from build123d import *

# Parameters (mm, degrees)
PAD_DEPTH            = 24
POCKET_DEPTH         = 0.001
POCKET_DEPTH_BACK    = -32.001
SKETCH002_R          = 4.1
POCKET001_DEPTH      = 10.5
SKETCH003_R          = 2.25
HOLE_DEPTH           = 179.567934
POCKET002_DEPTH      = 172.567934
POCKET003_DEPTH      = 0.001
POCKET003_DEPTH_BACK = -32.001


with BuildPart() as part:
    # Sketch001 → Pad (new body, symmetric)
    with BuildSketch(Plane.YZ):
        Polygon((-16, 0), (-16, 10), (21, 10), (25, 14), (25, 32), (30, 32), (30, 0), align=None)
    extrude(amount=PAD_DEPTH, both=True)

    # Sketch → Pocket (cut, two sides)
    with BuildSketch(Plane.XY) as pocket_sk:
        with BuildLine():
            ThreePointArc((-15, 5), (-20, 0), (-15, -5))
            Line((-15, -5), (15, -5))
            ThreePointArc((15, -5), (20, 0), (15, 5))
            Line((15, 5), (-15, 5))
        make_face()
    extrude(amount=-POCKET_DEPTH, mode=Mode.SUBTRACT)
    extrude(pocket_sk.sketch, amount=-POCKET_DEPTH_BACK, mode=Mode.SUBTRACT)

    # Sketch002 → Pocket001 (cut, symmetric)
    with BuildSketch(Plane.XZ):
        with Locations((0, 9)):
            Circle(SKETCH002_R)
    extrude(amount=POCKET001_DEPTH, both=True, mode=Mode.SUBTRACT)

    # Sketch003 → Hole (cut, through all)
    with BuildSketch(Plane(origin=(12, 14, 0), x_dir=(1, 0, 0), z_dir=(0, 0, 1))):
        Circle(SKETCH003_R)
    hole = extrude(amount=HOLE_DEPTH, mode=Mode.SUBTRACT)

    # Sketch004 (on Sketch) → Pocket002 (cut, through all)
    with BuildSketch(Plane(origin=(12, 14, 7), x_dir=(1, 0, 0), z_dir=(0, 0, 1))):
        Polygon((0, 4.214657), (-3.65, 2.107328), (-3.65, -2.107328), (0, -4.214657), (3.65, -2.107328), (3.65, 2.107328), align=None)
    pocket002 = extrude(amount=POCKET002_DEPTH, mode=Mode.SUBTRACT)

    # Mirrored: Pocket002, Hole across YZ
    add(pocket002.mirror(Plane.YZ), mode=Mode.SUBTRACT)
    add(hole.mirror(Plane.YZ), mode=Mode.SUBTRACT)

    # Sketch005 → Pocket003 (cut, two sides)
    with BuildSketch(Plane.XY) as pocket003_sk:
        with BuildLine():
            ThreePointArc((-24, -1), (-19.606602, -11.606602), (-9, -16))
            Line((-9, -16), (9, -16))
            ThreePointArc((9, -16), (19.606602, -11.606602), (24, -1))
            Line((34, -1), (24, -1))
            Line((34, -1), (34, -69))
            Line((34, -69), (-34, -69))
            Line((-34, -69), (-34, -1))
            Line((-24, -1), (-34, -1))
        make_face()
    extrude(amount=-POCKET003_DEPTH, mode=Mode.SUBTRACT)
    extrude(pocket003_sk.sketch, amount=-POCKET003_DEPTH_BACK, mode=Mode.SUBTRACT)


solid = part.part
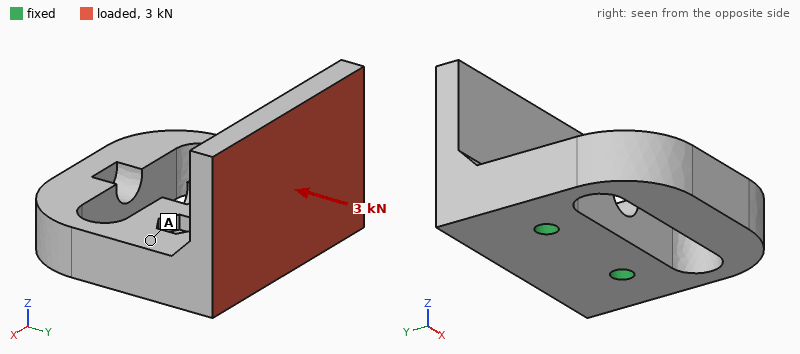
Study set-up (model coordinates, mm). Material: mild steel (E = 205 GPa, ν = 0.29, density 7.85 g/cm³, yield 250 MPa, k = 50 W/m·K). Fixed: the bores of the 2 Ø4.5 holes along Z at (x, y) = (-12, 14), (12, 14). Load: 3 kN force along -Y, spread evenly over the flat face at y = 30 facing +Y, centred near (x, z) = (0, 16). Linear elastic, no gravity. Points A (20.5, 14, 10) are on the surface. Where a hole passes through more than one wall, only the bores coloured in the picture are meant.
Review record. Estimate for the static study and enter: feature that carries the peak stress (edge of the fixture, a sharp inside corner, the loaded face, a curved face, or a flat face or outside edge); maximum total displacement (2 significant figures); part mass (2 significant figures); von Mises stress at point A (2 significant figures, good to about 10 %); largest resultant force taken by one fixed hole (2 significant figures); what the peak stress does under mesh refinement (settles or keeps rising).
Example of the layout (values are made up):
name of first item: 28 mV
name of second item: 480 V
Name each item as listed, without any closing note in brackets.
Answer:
feature that carries the peak stress: edge of the fixture
maximum total displacement: 49 µm
part mass: 170 g
von Mises stress at point A: 25 MPa
largest resultant force taken by one fixed hole: 1.5 kN
what the peak stress does under mesh refinement: keeps rising
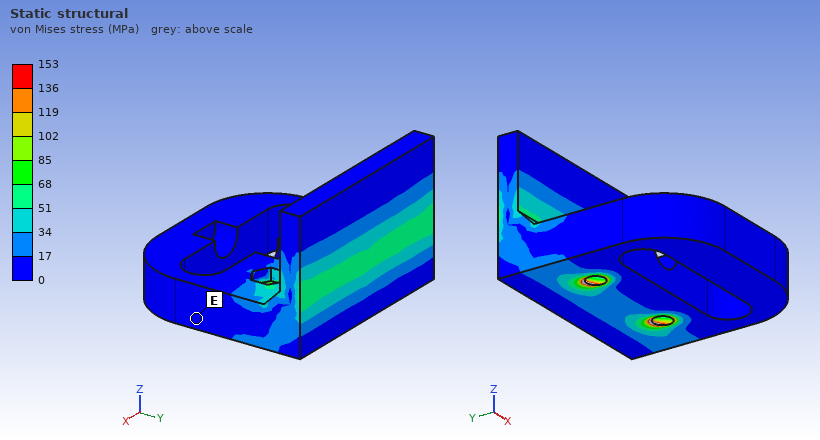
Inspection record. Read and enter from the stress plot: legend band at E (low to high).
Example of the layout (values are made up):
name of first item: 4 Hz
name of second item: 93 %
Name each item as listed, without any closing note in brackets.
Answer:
legend band at E: 0 to 17 MPa
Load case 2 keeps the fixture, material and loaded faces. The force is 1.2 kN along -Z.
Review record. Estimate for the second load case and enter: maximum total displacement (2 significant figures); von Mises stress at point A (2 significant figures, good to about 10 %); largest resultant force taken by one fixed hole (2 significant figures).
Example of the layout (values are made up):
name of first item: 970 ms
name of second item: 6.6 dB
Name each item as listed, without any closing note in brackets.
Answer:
maximum total displacement: 15 µm
von Mises stress at point A: 11 MPa
largest resultant force taken by one fixed hole: 600 N
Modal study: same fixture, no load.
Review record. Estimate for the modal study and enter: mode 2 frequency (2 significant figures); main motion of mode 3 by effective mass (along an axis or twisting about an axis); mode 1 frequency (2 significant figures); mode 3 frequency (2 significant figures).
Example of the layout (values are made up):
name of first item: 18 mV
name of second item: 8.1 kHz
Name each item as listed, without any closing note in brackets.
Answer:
mode 2 frequency: 6200 Hz
main motion of mode 3 by effective mass: along X
mode 1 frequency: 4300 Hz
mode 3 frequency: 8100 Hz
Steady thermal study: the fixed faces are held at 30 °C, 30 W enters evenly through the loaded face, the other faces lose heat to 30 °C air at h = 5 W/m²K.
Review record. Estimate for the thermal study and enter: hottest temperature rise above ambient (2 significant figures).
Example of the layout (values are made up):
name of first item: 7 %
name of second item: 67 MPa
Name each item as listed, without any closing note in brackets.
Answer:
hottest temperature rise above ambient: 39 K
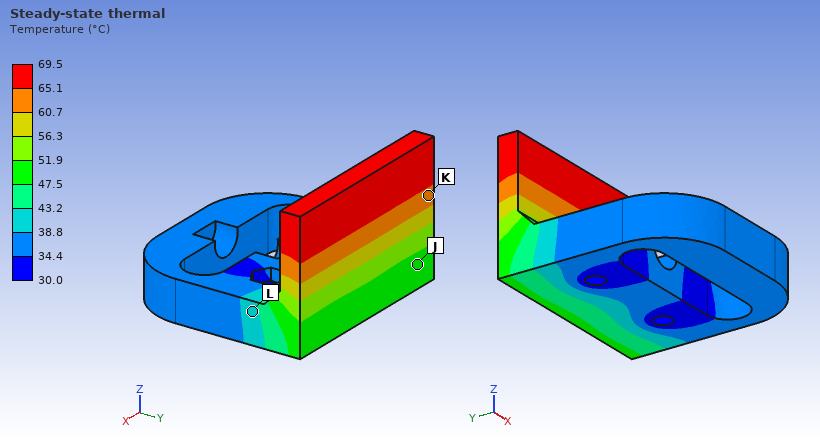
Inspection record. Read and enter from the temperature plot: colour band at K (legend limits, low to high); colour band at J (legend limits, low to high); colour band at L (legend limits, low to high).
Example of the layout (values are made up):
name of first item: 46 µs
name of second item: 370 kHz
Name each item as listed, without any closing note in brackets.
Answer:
colour band at K: 60.7 to 65.1 °C
colour band at J: 47.5 to 51.9 °C
colour band at L: 38.8 to 43.2 °C
